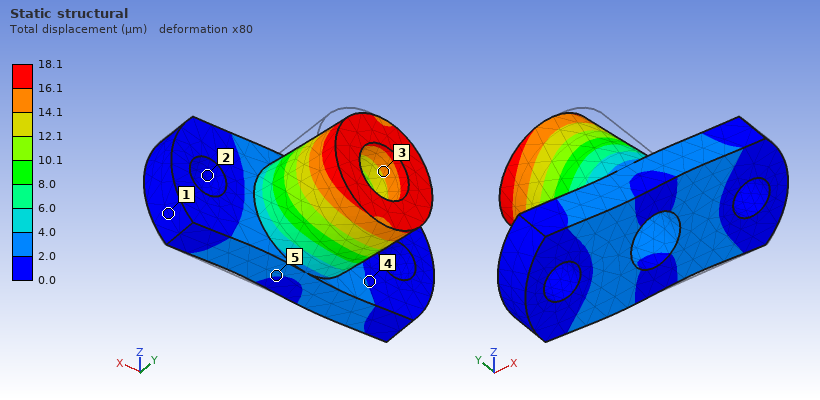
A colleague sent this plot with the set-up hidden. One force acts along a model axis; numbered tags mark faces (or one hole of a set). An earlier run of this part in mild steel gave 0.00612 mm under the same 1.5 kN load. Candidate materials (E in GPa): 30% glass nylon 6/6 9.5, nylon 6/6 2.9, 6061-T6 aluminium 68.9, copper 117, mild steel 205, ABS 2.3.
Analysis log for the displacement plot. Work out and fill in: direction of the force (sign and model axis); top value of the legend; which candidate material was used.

-X
18.1 µm
6061-T6 aluminium
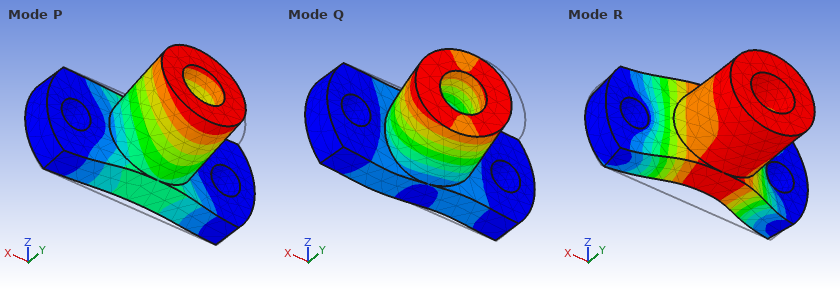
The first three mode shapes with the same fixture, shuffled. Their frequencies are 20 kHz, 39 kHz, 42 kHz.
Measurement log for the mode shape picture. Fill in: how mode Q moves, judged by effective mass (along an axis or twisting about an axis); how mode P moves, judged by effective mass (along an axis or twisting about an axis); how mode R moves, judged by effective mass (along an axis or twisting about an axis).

along X
along Z
along Y
